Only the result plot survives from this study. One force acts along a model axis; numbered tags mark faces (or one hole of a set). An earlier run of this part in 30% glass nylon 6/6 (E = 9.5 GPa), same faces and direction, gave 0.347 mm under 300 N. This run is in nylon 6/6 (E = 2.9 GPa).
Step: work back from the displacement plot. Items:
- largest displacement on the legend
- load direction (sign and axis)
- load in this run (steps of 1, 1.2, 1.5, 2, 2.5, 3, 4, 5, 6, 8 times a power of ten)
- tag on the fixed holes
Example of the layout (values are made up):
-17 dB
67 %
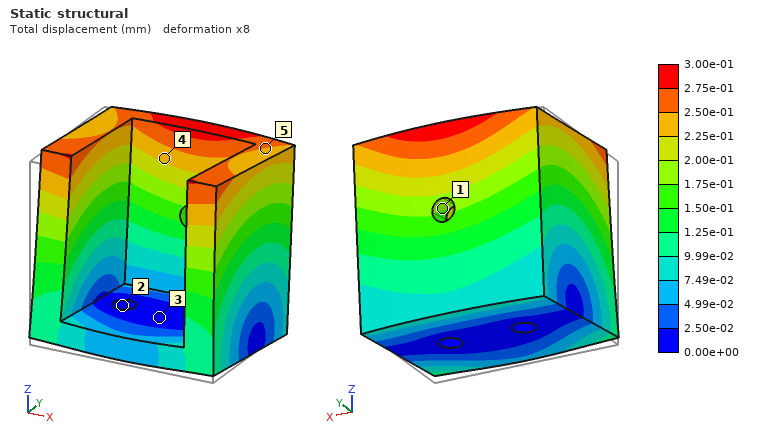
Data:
3.00e-01 mm
+Y
80 N
2
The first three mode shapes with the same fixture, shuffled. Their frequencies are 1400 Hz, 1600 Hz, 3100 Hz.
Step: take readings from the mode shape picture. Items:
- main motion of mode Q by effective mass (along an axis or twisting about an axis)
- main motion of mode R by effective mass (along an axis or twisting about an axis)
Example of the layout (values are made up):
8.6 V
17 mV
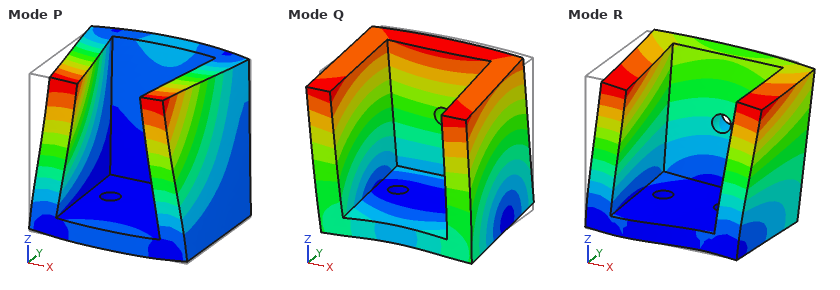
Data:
along Y
along X
